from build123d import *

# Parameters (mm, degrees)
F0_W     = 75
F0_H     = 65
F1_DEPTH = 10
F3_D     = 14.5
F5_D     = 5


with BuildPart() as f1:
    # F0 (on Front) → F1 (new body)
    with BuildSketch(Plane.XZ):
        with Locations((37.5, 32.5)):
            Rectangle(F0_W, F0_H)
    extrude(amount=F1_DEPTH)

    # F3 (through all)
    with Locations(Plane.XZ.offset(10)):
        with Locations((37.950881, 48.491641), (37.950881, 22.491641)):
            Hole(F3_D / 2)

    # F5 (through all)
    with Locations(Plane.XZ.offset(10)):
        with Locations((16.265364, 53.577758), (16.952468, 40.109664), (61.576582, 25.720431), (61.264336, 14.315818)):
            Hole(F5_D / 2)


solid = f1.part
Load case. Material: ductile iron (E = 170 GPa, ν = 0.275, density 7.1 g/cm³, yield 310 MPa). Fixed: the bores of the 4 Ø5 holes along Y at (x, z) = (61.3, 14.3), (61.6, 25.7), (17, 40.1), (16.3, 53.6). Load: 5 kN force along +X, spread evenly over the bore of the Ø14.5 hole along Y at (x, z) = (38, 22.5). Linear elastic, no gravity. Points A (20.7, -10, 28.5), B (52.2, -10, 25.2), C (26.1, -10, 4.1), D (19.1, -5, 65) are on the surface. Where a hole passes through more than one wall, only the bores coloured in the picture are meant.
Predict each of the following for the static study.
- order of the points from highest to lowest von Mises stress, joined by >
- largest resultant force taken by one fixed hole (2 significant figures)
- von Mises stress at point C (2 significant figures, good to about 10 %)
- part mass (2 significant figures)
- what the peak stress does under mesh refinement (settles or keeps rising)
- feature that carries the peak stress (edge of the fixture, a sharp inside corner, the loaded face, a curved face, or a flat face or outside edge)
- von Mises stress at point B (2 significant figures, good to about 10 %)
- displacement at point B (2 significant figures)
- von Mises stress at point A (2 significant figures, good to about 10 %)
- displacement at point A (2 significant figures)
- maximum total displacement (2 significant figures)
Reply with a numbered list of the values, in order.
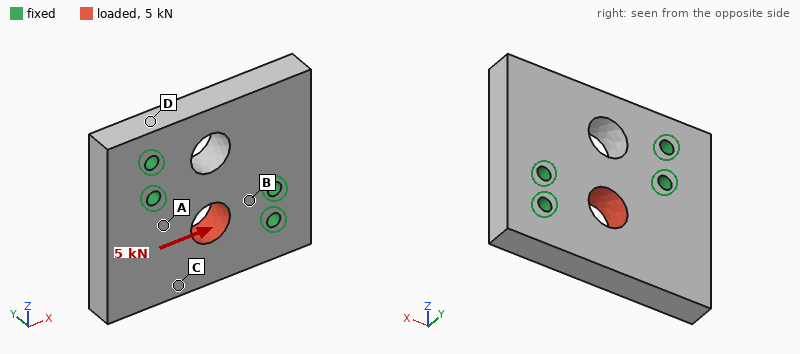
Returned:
1. B > A > C > D
2. 1.9 kN
3. 4.7 MPa
4. 320 g
5. keeps rising
6. edge of the fixture
7. 12 MPa
8. 0.56 µm
9. 7.8 MPa
10. 1.2 µm
11. 2.3 µm
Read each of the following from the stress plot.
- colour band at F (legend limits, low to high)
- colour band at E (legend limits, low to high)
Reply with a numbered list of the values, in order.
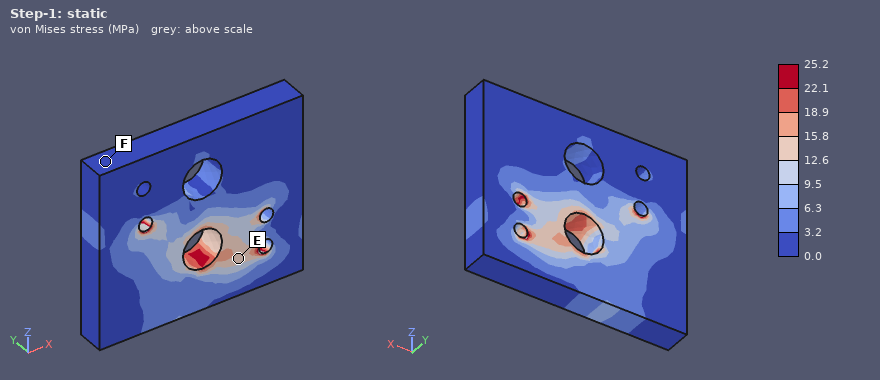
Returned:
1. 0.0 to 3.2 MPa
2. 12.6 to 15.8 MPa
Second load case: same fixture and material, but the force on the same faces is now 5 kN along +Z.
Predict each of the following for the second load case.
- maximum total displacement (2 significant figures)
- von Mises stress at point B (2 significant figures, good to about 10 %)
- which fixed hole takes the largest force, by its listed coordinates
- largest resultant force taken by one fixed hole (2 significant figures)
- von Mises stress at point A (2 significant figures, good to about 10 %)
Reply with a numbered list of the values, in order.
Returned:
1. 2.7 µm
2. 11 MPa
3. (17, 40.1)
4. 1.8 kN
5. 11 MPa
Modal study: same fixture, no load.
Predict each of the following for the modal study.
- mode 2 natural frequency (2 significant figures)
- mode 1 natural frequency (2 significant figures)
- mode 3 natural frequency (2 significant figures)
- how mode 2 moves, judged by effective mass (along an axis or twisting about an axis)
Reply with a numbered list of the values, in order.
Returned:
1. 6200 Hz
2. 5500 Hz
3. 13 kHz
4. along Y
